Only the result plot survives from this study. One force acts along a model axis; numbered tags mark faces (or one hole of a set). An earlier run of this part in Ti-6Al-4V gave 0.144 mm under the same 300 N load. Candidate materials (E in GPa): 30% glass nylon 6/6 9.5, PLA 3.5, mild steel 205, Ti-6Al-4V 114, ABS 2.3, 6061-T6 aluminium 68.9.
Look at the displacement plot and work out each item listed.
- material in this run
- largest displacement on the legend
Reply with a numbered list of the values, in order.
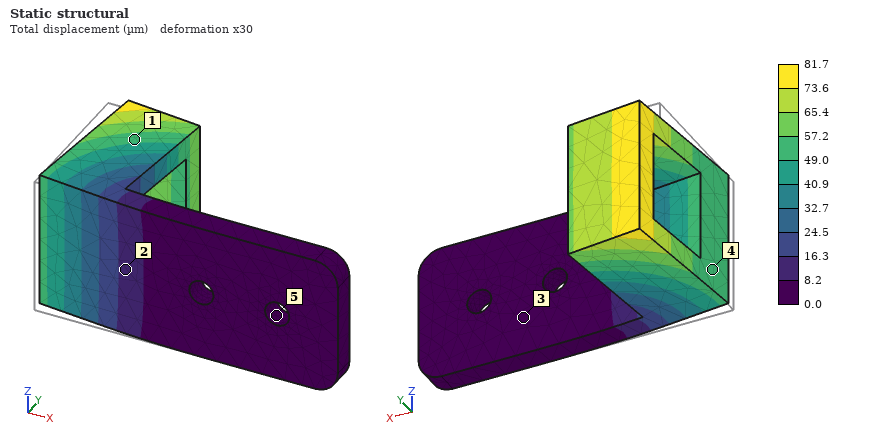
1. mild steel
2. 81.7 µm
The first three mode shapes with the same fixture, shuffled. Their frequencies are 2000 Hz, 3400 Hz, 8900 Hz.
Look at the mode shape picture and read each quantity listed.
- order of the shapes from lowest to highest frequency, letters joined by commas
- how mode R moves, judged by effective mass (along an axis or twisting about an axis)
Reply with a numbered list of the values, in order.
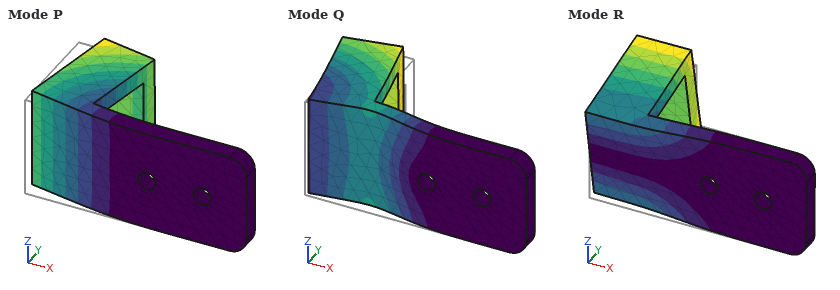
1. P, R, Q
2. along Z
